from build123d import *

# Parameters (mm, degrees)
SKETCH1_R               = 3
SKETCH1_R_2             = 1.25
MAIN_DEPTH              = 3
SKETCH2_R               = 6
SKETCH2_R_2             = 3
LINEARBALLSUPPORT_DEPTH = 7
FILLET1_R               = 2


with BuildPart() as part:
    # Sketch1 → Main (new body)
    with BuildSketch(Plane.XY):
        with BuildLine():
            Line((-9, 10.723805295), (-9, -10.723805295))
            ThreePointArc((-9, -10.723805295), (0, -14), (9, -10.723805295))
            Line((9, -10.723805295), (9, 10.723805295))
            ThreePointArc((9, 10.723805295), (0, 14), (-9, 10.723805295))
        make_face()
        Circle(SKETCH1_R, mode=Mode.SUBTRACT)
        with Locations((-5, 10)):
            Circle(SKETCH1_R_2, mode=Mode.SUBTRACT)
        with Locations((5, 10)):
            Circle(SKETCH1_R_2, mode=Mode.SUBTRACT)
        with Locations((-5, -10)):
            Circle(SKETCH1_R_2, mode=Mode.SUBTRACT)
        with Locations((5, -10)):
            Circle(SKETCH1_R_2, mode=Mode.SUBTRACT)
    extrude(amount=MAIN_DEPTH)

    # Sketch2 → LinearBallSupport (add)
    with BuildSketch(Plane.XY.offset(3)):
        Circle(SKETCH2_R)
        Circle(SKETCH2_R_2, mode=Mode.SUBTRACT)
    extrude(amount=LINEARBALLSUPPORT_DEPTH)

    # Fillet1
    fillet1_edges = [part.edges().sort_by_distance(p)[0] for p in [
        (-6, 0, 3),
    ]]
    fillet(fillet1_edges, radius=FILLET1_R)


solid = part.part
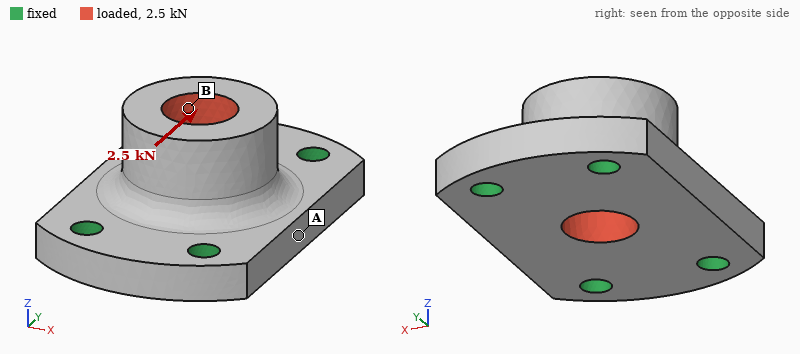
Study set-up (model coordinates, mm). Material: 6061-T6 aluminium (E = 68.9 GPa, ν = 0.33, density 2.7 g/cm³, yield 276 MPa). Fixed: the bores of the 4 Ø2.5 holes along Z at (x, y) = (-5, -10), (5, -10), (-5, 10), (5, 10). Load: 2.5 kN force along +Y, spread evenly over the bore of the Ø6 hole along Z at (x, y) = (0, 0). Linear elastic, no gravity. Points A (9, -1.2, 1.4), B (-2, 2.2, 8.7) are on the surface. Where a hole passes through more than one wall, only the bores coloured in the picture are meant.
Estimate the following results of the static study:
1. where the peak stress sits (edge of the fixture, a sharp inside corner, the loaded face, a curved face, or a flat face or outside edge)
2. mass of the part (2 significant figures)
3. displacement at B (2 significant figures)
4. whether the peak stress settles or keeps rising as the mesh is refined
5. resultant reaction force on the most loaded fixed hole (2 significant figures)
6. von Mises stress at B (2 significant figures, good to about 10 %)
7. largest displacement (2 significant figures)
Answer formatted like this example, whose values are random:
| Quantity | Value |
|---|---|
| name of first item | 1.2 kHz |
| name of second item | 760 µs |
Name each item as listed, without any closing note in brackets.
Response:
| Quantity | Value |
|---|---|
| where the peak stress sits | edge of the fixture |
| mass of the part | 5.1 g |
| displacement at B | 11 µm |
| whether the peak stress settles or keeps rising as the mesh is refined | keeps rising |
| resultant reaction force on the most loaded fixed hole | 700 N |
| von Mises stress at B | 28 MPa |
| largest displacement | 13 µm |
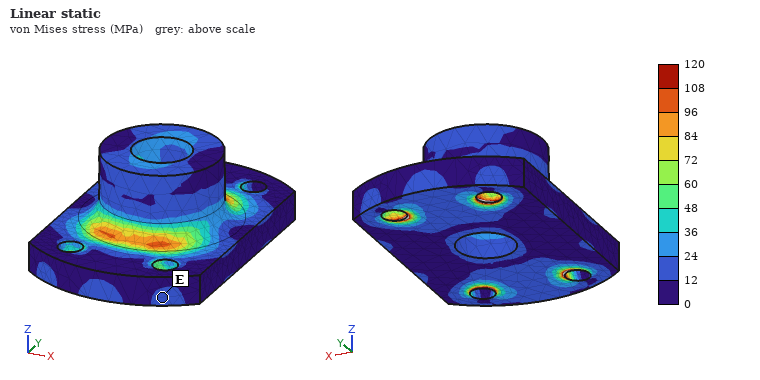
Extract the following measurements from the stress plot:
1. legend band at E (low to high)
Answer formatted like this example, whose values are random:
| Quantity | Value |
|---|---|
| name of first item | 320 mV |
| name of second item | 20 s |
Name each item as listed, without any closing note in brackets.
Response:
| Quantity | Value |
|---|---|
| legend band at E | 12 to 24 MPa |
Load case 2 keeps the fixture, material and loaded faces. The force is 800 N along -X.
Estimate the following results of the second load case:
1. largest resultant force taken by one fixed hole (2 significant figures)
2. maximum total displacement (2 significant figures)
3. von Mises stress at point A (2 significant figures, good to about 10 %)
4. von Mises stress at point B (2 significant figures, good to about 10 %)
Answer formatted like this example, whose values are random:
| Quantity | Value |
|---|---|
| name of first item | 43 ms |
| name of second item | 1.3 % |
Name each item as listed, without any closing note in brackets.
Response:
| Quantity | Value |
|---|---|
| largest resultant force taken by one fixed hole | 270 N |
| maximum total displacement | 9.4 µm |
| von Mises stress at point A | 13 MPa |
| von Mises stress at point B | 9.4 MPa |
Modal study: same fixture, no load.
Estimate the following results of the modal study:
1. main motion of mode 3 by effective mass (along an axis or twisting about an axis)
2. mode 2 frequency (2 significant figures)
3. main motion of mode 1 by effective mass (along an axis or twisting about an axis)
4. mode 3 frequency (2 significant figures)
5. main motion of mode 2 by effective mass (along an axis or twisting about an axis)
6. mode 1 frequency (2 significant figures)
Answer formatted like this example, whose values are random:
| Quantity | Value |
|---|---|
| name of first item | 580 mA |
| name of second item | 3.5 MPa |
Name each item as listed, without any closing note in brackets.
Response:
| Quantity | Value |
|---|---|
| main motion of mode 3 by effective mass | along Y |
| mode 2 frequency | 35 kHz |
| main motion of mode 1 by effective mass | along X |
| mode 3 frequency | 50 kHz |
| main motion of mode 2 by effective mass | along Z |
| mode 1 frequency | 30 kHz |
